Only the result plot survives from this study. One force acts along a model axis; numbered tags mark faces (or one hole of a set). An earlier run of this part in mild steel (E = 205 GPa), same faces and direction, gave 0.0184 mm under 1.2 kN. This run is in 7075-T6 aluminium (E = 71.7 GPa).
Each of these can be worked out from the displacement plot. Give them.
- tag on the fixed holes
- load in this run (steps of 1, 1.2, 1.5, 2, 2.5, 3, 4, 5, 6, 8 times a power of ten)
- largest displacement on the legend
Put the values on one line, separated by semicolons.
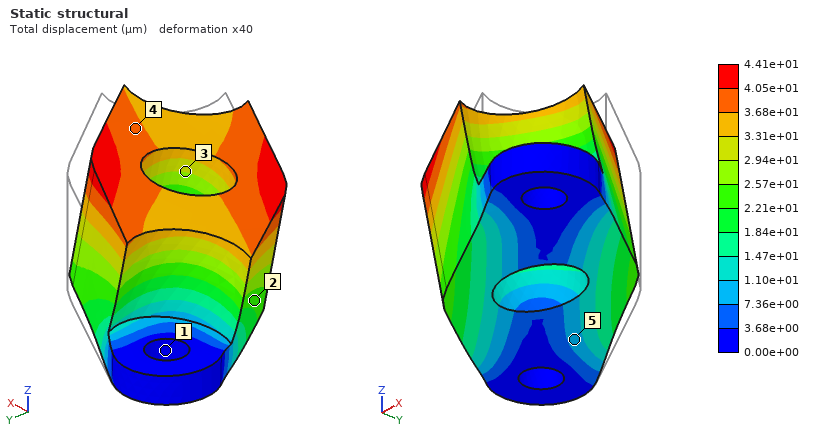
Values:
1; 1 kN; 4.41e+01 µm
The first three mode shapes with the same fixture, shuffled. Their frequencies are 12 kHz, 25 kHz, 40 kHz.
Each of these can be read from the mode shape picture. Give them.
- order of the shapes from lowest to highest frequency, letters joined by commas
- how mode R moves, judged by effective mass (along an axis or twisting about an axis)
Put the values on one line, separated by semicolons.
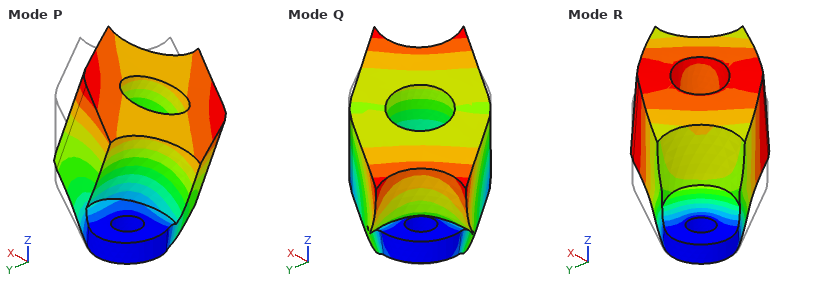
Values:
P, R, Q; along Z
